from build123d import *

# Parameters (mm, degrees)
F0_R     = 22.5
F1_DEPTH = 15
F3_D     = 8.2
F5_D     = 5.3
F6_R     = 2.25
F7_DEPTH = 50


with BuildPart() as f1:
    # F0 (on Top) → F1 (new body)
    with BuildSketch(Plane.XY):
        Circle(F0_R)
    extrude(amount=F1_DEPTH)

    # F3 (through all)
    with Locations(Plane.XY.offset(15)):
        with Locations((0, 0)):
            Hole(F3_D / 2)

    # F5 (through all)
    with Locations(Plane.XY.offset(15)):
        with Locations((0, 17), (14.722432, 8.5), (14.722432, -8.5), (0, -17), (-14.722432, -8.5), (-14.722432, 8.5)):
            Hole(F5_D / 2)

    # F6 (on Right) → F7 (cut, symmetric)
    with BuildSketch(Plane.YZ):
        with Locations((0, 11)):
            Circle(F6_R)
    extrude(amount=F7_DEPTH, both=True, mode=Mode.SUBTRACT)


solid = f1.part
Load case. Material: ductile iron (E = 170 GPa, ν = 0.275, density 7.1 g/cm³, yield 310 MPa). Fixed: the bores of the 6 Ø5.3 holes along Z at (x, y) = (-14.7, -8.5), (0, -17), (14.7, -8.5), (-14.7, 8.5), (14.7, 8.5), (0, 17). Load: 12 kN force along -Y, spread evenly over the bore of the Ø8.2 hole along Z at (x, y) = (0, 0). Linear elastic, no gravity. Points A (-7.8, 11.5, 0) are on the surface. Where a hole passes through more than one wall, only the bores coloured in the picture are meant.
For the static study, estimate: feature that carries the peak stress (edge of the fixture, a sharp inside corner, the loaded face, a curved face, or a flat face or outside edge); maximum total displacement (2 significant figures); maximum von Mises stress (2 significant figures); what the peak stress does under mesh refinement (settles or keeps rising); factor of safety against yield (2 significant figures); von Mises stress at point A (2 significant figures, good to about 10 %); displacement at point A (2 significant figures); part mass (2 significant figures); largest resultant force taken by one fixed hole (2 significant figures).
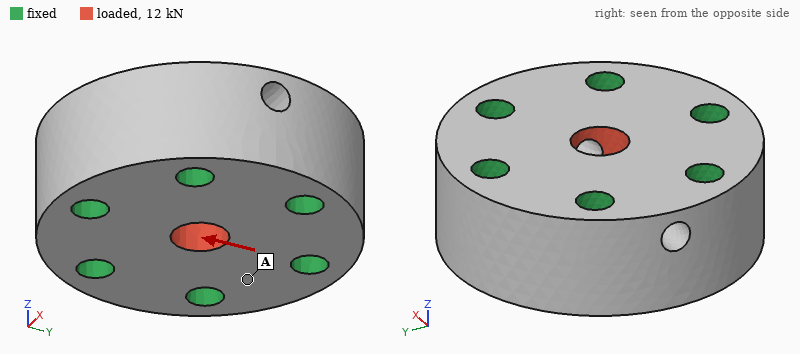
the loaded face
1.9 µm
82 MPa
settles
3.8
7.7 MPa
0.54 µm
150 g
3.4 kN
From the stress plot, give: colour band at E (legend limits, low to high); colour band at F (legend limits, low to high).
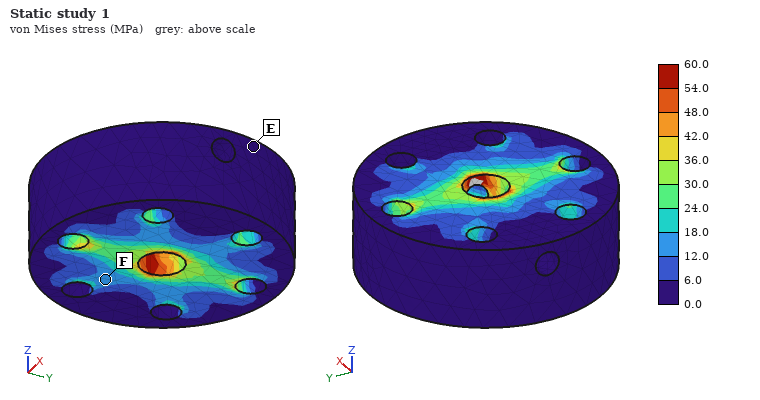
0.0 to 6.0 MPa
12.0 to 18.0 MPa
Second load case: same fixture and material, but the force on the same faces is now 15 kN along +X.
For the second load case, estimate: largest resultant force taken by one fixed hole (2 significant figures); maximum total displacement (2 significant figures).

3.5 kN
2.4 µm
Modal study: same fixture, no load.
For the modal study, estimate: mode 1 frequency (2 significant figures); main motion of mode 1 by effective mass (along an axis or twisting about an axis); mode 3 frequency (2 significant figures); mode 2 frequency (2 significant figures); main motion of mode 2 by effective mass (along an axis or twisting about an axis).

63 kHz
along Z
86 kHz
81 kHz
twisting about X
